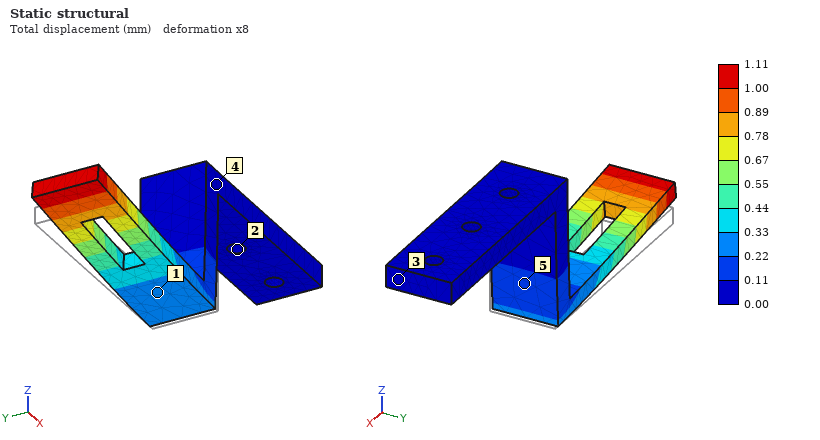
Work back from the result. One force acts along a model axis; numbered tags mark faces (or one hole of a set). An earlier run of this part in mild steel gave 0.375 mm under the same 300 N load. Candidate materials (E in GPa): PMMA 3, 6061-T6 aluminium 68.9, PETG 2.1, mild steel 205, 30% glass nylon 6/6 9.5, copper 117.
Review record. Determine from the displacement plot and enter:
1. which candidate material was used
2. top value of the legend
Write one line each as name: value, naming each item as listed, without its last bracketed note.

which candidate material was used: 6061-T6 aluminium
top value of the legend: 1.11 mm
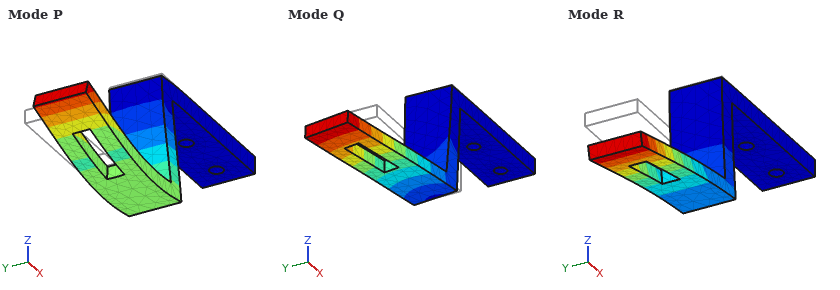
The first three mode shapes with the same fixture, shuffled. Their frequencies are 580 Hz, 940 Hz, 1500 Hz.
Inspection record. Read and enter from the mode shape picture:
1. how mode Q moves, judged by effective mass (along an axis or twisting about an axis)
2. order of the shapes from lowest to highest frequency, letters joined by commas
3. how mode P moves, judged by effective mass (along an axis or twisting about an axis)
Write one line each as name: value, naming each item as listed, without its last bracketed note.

how mode Q moves, judged by effective mass: along Y
order of the shapes from lowest to highest frequency, letters joined by commas: R, Q, P
how mode P moves, judged by effective mass: along X
